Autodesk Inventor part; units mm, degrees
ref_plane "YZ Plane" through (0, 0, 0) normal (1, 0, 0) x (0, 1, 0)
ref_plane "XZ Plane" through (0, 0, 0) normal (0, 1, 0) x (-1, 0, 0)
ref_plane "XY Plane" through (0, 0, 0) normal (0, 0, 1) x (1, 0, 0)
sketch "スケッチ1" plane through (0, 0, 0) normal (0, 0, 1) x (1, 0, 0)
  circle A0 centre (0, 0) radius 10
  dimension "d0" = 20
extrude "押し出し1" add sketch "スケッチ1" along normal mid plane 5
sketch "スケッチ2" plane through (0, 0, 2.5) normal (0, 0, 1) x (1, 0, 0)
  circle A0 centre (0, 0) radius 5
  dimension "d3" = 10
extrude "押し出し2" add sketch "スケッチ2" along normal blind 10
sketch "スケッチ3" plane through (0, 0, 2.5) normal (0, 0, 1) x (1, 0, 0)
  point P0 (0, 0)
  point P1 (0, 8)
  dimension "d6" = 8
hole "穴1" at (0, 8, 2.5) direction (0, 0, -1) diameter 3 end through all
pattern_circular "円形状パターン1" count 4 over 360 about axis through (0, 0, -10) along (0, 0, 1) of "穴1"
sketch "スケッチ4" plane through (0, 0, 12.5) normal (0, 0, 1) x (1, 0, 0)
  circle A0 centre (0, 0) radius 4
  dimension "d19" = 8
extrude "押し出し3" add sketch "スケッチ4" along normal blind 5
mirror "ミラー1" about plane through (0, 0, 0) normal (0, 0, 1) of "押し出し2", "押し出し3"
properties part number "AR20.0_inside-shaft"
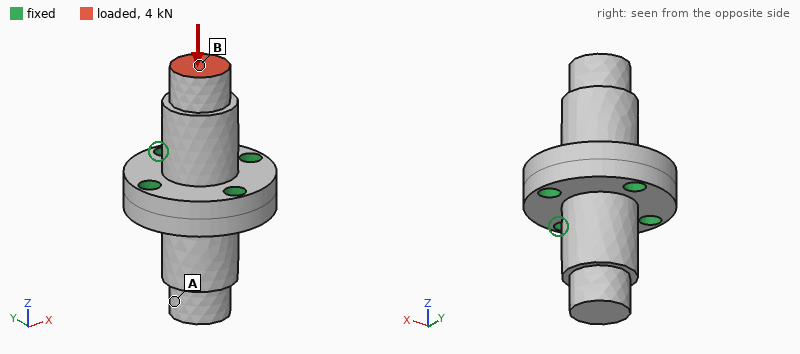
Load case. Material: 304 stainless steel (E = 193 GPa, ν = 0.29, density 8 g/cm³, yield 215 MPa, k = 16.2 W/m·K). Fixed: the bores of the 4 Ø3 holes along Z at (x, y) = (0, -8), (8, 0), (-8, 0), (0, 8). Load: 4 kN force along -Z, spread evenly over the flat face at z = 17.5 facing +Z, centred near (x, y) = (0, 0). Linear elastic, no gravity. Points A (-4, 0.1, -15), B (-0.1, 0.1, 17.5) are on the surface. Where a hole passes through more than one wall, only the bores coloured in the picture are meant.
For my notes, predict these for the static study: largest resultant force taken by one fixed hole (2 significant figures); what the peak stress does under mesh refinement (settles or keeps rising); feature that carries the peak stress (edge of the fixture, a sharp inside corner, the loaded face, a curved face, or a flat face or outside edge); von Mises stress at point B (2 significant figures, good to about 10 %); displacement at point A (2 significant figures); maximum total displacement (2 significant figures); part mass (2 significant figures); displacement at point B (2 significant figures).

1.0 kN
keeps rising
edge of the fixture
79 MPa
1.2 µm
6.6 µm
28 g
6.5 µm
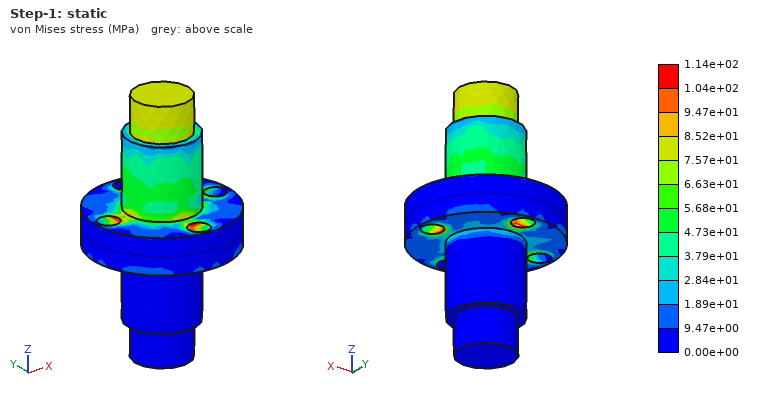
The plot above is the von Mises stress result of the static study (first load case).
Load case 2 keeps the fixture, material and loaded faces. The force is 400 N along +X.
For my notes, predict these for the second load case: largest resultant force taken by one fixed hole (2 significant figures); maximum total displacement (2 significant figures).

480 N
9.7 µm
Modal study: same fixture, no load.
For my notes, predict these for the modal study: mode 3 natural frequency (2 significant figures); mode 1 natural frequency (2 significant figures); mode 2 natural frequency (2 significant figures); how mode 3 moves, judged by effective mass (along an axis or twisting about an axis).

25 kHz
21 kHz
21 kHz
along X
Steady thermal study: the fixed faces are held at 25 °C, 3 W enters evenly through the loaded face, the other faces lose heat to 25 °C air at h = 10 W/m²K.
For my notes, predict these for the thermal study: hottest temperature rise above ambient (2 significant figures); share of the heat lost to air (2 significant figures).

49 K
4.5 %
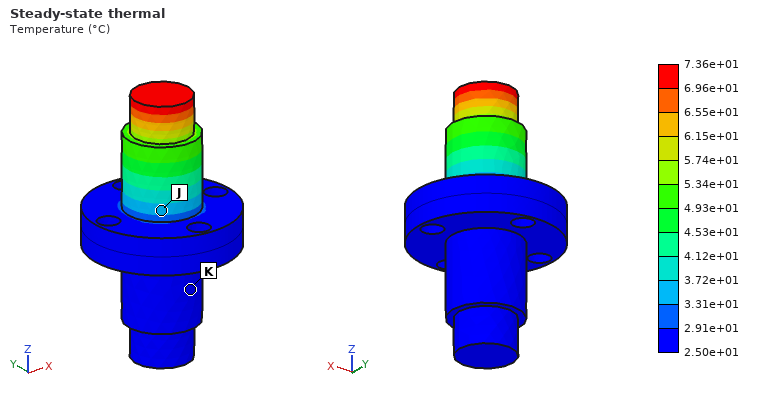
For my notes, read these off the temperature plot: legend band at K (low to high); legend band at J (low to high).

2.50e+01 to 2.91e+01 °C
3.31e+01 to 3.72e+01 °C
